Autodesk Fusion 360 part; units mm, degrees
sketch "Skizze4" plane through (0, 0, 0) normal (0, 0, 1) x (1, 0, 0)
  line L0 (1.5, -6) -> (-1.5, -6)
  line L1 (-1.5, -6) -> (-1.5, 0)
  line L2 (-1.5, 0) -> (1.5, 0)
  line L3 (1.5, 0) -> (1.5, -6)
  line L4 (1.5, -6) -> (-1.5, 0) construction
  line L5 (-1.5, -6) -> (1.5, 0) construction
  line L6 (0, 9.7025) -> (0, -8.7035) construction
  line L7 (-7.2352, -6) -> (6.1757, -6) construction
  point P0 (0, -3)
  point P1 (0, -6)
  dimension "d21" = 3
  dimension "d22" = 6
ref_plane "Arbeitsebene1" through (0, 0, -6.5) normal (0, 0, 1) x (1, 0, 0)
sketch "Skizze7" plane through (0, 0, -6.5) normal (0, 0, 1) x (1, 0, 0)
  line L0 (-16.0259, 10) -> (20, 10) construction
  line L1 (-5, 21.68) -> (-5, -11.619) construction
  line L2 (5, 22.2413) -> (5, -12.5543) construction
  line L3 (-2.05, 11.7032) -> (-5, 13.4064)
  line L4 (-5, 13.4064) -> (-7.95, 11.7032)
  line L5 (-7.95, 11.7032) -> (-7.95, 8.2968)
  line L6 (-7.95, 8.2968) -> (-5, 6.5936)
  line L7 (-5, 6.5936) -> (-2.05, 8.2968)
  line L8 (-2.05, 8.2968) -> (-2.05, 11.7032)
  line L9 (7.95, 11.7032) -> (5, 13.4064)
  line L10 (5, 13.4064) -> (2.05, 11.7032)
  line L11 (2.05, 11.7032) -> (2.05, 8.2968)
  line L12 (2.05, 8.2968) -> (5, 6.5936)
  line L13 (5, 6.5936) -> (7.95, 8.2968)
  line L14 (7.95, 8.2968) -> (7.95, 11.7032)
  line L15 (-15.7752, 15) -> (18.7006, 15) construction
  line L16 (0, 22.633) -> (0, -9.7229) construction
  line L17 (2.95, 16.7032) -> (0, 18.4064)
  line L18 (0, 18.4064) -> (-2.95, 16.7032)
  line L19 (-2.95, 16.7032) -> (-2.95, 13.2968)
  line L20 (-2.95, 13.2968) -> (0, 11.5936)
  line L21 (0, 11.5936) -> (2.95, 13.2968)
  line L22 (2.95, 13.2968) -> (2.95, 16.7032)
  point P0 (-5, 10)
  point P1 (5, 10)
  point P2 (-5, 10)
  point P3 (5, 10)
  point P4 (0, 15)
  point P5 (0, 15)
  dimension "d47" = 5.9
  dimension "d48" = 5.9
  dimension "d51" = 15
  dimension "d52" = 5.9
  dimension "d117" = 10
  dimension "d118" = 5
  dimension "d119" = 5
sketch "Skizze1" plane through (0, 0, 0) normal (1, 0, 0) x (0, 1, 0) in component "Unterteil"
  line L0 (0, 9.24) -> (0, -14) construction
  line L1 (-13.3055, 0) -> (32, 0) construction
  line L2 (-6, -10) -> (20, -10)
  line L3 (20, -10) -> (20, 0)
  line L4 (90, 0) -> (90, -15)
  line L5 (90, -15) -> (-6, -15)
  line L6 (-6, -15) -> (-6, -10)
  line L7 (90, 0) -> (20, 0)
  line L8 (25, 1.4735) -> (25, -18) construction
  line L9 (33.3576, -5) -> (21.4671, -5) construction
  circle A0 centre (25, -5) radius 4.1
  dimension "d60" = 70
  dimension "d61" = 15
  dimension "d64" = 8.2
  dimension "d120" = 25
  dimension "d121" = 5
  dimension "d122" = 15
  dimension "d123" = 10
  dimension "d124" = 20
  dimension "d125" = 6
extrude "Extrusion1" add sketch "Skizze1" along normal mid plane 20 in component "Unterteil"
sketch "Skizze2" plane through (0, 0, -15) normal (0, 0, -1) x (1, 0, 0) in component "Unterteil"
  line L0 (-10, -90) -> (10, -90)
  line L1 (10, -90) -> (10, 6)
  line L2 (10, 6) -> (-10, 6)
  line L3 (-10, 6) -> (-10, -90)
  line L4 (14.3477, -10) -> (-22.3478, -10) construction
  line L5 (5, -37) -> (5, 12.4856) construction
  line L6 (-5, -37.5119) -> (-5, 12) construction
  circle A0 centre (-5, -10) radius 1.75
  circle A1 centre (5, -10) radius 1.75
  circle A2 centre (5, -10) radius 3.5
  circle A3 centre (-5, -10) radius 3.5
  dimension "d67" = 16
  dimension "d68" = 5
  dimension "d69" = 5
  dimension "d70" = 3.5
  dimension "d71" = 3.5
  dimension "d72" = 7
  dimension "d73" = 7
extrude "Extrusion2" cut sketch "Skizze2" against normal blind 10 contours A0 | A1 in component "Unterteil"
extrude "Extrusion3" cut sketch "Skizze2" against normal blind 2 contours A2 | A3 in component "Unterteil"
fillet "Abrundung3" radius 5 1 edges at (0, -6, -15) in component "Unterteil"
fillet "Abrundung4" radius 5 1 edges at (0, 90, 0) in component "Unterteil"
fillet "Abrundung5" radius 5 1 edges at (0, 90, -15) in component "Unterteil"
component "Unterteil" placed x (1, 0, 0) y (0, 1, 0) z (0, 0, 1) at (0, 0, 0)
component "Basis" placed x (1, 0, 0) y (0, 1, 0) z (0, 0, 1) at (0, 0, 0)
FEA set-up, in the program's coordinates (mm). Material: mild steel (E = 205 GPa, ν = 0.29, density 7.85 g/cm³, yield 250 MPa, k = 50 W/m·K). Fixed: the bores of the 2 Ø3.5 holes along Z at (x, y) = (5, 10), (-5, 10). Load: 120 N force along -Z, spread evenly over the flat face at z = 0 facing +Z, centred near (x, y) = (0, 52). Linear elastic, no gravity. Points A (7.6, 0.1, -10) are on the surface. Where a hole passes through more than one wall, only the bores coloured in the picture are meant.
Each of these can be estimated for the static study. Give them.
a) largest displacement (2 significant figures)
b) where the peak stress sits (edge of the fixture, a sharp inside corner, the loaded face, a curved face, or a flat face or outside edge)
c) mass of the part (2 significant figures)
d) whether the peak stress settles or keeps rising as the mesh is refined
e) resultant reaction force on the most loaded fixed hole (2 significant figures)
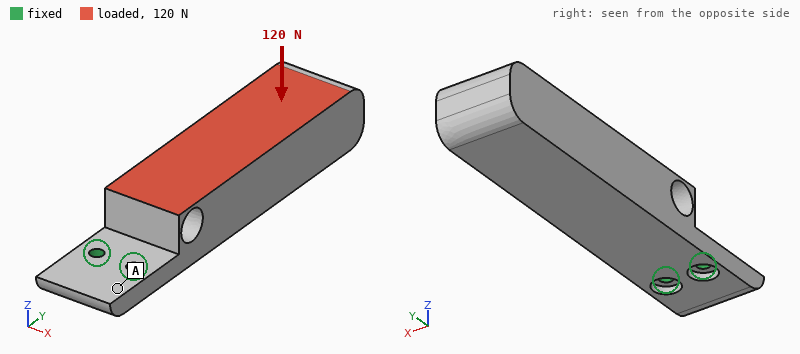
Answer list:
0.15 mm
edge of the fixture
170 g
keeps rising
66 N
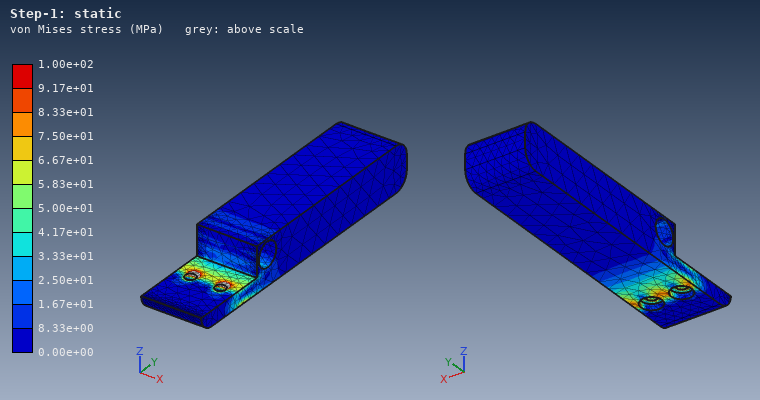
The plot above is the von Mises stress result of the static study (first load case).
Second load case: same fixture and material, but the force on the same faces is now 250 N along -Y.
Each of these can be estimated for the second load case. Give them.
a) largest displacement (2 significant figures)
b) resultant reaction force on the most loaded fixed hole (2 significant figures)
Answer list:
0.10 mm
130 N
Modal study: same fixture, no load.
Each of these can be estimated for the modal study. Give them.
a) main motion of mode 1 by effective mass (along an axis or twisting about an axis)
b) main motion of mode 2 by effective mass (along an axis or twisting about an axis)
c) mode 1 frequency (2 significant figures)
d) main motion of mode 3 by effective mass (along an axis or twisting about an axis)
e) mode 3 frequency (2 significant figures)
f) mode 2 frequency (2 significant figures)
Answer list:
along Z
along X
420 Hz
twisting about Y
4000 Hz
1400 Hz
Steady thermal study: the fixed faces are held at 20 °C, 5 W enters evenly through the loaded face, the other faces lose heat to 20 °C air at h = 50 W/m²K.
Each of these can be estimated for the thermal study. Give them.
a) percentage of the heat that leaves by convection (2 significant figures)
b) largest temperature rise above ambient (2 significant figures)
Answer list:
51 %
14 K
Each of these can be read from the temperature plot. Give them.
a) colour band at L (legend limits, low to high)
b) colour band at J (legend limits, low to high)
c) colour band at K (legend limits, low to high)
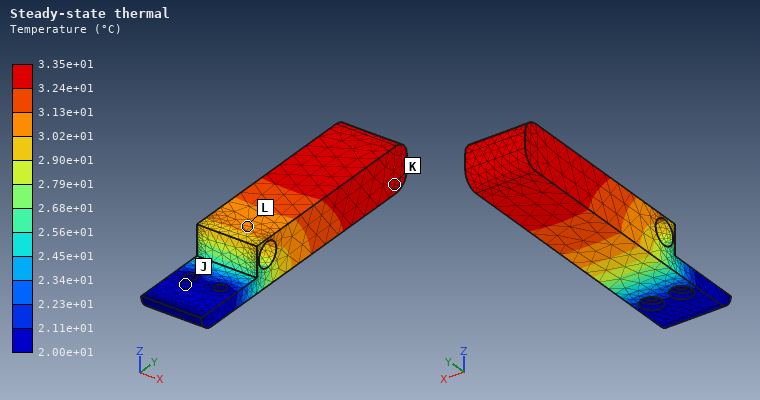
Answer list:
3.02e+01 to 3.13e+01 °C
2.00e+01 to 2.11e+01 °C
3.24e+01 to 3.35e+01 °C
